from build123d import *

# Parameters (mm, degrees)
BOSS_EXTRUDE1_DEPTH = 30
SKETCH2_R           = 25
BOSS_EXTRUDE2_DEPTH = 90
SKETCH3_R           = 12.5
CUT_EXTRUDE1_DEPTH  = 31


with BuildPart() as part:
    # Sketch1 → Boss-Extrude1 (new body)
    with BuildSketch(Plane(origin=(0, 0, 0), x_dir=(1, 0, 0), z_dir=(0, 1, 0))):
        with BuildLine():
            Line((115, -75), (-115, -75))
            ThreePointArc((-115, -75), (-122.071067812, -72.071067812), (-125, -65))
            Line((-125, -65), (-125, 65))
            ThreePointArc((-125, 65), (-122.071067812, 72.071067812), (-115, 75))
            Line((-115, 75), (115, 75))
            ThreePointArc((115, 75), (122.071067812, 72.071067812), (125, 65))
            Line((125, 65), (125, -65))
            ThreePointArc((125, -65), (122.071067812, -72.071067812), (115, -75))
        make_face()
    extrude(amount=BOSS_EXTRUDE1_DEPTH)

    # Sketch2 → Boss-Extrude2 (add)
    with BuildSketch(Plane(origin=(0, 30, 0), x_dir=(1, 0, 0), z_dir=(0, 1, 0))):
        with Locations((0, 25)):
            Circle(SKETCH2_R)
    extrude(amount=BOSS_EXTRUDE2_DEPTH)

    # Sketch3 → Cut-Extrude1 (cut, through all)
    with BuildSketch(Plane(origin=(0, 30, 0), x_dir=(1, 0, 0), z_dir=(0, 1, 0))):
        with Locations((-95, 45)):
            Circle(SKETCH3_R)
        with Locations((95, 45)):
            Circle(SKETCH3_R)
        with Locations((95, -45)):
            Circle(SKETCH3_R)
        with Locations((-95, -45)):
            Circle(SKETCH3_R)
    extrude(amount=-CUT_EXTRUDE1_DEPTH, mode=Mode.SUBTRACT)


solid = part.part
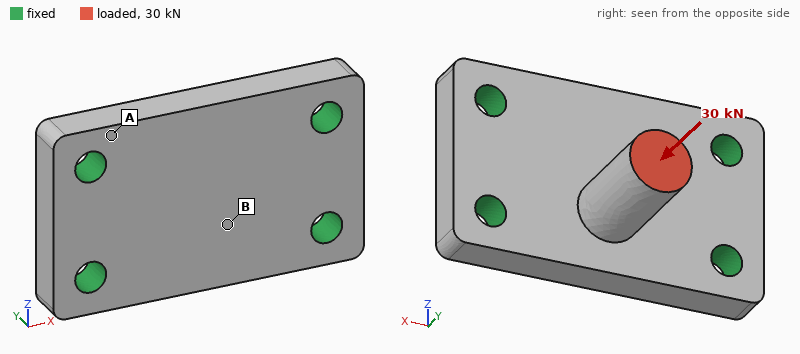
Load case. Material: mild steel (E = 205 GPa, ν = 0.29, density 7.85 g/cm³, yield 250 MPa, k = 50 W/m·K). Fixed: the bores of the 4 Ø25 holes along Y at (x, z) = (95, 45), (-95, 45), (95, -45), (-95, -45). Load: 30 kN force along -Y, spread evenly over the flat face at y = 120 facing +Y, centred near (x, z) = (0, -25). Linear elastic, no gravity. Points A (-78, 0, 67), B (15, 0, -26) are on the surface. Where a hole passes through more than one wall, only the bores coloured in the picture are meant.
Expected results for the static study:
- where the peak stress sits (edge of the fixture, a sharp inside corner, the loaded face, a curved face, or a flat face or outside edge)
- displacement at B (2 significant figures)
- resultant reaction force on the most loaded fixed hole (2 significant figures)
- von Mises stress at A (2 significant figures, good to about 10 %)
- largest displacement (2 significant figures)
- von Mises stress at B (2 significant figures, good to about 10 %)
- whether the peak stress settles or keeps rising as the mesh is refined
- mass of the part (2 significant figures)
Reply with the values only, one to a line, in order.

edge of the fixture
18 µm
11 kN
8.1 MPa
28 µm
24 MPa
keeps rising
9.7 kg
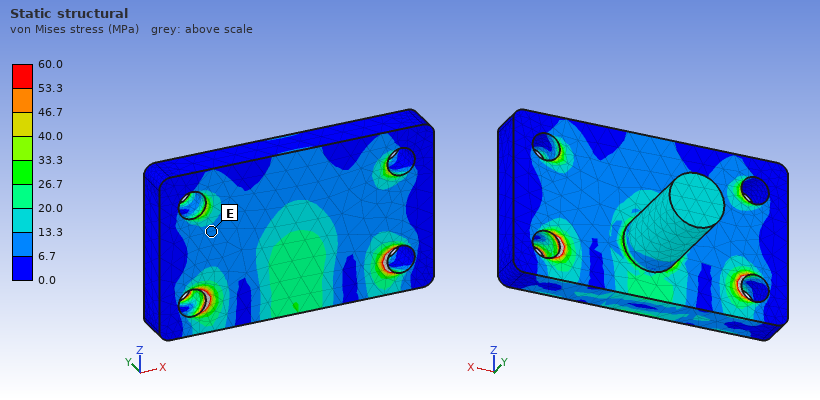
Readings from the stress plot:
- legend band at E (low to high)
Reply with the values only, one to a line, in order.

6.7 to 13.3 MPa
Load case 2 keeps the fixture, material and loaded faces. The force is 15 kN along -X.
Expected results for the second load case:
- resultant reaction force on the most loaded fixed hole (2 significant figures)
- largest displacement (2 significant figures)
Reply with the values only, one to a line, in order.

10 kN
0.12 mm
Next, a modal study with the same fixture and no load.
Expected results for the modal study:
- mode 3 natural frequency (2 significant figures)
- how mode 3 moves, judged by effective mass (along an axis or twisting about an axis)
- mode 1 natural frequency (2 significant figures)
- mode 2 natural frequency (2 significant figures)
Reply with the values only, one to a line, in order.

3400 Hz
along Y
2300 Hz
2700 Hz
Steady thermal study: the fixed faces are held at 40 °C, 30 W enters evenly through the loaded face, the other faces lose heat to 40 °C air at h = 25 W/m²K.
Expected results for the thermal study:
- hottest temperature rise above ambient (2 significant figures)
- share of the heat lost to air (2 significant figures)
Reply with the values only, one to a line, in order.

31 K
32 %
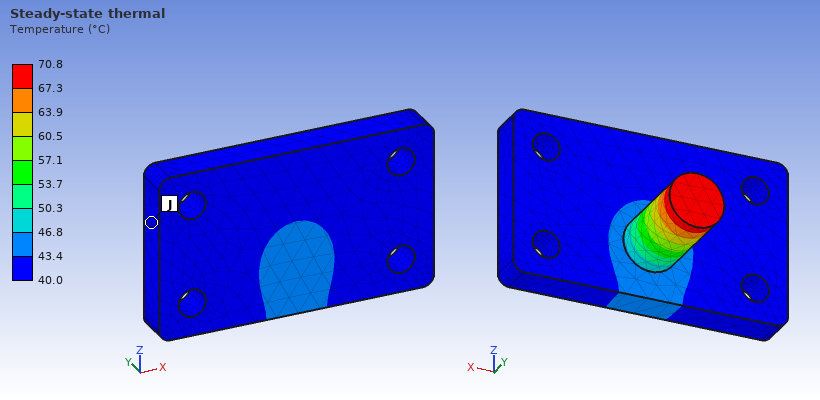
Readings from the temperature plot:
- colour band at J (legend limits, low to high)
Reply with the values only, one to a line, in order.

40.0 to 43.4 °C
